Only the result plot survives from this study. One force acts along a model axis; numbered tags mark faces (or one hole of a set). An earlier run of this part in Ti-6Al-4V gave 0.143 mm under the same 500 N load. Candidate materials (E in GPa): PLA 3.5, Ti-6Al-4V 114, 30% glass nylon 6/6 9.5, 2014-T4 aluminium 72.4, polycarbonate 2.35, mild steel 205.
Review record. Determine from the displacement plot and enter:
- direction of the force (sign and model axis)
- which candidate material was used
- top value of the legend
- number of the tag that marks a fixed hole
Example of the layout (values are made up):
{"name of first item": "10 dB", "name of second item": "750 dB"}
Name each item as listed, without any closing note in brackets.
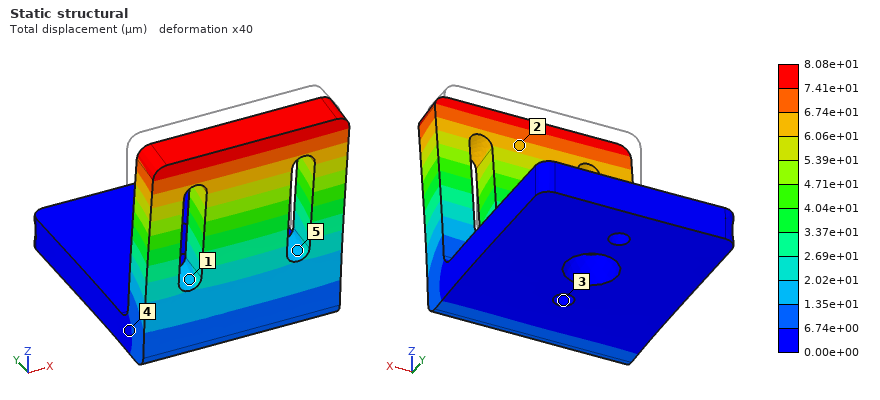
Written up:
{"direction of the force": "-Y", "which candidate material was used": "mild steel", "top value of the legend": "8.08e+01 µm", "number of the tag that marks a fixed hole": "3"}
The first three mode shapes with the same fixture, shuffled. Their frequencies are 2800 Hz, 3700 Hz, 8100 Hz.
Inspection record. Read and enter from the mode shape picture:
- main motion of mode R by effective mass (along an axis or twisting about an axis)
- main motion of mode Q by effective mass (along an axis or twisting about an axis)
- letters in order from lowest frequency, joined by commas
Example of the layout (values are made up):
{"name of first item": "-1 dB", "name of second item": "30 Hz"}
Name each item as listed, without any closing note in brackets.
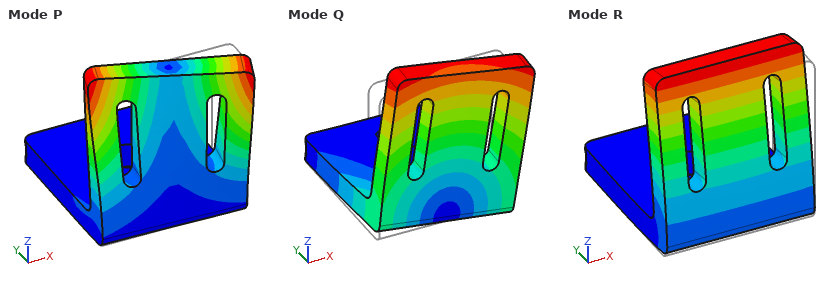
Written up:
{"main motion of mode R by effective mass": "along Y", "main motion of mode Q by effective mass": "along X", "letters in order from lowest frequency, joined by commas": "R, Q, P"}
